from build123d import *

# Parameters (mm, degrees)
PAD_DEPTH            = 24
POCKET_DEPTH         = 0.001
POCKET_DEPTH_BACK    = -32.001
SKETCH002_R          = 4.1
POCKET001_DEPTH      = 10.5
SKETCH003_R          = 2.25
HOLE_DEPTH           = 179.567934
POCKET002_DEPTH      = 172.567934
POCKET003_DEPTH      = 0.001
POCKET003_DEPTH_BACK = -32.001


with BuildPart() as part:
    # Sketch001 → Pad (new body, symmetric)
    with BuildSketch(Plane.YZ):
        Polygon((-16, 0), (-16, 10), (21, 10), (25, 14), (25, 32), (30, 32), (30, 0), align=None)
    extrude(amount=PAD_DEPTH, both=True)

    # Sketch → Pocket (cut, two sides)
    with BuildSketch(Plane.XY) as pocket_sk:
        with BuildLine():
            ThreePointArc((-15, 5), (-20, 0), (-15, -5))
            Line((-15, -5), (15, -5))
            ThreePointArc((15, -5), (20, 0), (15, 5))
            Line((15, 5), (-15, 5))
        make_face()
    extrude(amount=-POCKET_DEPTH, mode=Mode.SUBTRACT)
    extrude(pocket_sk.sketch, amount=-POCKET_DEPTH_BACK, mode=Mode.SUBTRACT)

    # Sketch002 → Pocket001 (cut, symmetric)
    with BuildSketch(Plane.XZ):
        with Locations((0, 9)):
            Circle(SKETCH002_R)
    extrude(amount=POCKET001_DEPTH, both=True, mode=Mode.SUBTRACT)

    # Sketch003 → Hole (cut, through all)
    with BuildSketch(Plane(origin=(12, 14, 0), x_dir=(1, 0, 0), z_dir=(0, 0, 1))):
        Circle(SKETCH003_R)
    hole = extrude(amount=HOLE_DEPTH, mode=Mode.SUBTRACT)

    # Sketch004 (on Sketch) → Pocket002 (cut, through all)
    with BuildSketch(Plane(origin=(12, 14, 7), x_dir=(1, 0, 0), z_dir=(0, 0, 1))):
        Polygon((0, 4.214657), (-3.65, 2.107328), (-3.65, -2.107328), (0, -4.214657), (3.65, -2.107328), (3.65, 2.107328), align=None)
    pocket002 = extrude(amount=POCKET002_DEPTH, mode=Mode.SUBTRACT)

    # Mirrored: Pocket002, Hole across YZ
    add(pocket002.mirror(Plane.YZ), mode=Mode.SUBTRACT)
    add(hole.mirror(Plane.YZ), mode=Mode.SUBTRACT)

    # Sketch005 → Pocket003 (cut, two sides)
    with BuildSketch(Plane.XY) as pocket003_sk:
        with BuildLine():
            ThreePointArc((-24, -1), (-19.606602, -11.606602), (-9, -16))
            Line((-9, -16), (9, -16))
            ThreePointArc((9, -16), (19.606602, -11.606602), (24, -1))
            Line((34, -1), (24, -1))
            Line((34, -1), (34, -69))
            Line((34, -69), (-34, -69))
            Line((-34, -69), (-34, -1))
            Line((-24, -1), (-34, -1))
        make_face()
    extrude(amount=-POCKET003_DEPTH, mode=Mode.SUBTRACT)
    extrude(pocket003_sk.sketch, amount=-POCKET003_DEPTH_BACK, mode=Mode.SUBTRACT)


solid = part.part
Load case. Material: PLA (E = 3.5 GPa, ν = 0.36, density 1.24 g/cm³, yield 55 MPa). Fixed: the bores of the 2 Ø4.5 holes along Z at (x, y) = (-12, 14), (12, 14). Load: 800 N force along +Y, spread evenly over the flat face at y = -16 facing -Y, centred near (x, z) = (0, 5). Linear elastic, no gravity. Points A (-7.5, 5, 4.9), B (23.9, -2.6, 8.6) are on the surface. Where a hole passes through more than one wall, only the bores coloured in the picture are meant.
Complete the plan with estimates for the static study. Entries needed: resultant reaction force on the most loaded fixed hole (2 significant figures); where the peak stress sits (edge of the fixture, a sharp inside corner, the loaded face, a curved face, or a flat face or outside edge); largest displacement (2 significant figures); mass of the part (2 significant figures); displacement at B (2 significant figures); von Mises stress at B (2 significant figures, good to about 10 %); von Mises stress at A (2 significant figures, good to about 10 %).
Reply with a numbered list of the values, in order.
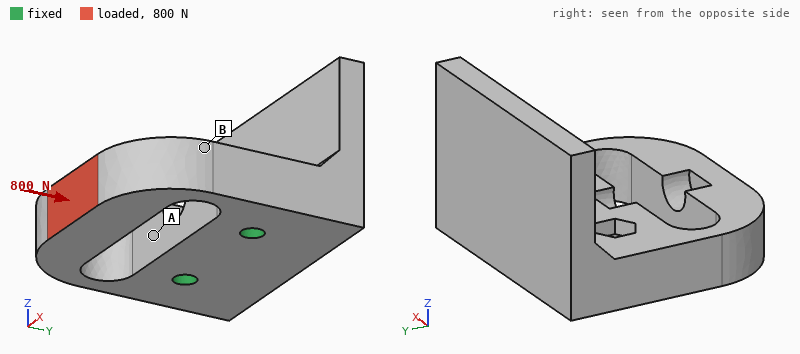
1. 450 N
2. a curved face
3. 0.42 mm
4. 27 g
5. 0.14 mm
6. 16 MPa
7. 5.8 MPa
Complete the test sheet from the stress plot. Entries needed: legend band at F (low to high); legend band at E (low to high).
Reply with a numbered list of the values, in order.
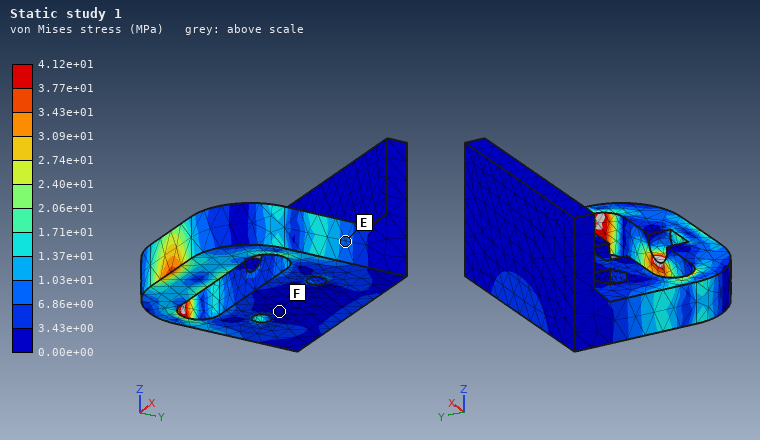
1. 0.00e+00 to 3.43e+00 MPa
2. 6.86e+00 to 1.03e+01 MPa
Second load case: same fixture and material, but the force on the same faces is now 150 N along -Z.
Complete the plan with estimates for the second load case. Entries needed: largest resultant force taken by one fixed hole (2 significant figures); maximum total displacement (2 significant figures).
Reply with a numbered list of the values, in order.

1. 80 N
2. 0.64 mm
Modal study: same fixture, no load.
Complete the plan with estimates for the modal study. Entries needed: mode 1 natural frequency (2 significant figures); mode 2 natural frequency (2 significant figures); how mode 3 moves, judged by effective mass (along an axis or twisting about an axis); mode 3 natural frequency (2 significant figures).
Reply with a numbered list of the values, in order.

1. 1400 Hz
2. 2100 Hz
3. along X
4. 2700 Hz
